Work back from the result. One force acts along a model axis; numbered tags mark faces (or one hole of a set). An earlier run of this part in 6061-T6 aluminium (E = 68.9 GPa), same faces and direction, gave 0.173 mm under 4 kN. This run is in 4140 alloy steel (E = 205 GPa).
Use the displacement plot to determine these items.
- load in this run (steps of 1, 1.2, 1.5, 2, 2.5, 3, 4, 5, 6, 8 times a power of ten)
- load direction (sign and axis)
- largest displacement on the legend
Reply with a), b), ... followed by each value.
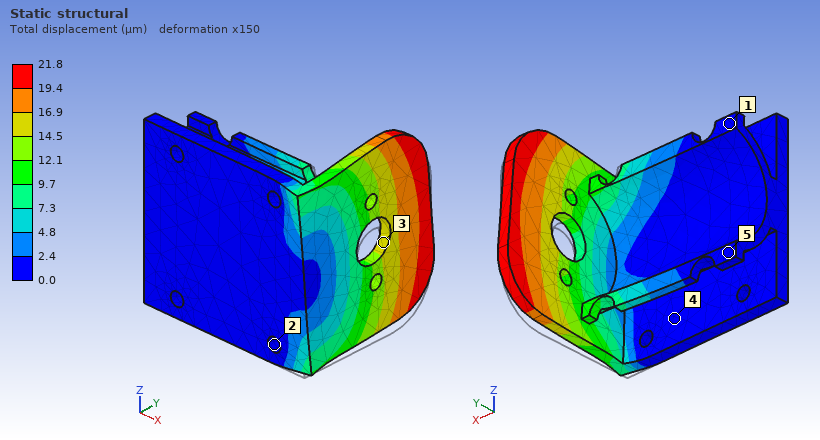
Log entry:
a) 1.5 kN
b) +Z
c) 21.8 µm
